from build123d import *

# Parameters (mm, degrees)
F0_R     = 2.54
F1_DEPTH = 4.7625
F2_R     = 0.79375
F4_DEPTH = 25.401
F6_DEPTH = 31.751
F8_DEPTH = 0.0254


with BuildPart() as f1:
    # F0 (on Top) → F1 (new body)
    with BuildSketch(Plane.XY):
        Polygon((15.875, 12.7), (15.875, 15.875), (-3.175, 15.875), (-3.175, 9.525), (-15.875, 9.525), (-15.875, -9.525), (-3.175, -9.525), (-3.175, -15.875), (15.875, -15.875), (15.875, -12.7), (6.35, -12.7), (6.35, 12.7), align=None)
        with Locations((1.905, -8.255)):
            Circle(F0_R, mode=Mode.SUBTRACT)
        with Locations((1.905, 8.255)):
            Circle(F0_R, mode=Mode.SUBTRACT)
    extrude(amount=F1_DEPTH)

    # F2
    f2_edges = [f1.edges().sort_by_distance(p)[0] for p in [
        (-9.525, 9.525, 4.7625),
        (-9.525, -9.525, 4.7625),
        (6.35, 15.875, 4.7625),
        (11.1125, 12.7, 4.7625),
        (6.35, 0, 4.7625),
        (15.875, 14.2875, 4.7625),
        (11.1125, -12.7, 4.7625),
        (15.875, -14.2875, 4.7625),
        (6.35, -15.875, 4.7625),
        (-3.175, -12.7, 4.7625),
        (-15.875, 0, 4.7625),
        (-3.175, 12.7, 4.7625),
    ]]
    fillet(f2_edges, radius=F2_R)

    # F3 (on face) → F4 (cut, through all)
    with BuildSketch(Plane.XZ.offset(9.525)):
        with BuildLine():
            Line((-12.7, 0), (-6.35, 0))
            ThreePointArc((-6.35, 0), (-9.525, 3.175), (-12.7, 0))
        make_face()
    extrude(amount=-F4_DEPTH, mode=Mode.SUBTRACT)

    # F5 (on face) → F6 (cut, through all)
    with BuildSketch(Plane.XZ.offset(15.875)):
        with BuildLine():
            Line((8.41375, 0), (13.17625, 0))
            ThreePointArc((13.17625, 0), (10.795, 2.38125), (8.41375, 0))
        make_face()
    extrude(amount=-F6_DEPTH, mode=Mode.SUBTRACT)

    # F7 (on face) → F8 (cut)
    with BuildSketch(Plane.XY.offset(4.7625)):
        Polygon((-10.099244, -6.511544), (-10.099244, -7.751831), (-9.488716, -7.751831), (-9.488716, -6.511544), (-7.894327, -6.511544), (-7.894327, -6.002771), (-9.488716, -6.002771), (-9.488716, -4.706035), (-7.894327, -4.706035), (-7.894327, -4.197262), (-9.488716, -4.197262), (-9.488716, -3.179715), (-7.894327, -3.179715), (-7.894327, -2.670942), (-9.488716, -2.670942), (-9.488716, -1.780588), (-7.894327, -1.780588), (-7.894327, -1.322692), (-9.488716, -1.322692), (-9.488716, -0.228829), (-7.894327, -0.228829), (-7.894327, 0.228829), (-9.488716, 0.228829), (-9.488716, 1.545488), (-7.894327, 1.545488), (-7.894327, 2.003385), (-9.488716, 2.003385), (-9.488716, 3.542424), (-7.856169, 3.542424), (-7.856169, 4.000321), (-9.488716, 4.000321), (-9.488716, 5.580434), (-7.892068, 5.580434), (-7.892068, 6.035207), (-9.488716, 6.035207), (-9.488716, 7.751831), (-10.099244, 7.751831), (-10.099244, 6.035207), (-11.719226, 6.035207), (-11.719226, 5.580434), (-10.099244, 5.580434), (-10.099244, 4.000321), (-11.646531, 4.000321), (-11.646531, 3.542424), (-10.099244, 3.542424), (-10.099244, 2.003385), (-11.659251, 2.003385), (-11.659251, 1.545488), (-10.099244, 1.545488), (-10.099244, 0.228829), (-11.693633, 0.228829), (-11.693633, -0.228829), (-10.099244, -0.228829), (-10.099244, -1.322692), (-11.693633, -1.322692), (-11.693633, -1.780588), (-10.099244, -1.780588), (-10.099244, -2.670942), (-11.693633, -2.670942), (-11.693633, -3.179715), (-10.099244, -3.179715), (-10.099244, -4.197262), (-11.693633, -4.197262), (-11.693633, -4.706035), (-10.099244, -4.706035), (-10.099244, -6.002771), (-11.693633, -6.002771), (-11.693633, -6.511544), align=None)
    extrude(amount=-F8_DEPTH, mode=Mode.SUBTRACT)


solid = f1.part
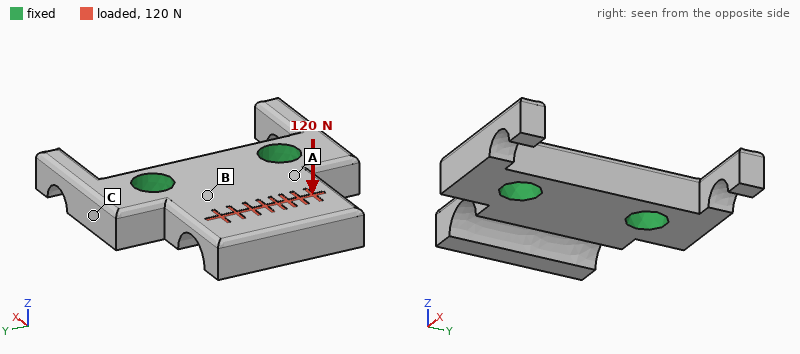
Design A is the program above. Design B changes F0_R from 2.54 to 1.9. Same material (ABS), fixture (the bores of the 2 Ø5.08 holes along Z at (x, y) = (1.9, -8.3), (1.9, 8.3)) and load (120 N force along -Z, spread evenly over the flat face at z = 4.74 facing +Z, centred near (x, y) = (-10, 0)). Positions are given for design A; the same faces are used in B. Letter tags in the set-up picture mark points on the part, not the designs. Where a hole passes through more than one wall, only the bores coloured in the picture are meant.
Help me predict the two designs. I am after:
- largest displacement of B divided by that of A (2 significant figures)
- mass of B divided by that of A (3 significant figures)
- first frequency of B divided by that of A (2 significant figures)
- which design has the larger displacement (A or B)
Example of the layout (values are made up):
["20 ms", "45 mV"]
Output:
["1.1", "1.04", "0.97", "B"]
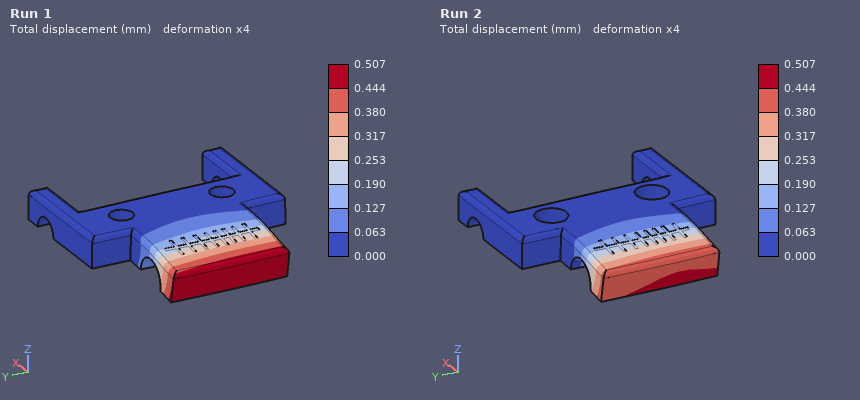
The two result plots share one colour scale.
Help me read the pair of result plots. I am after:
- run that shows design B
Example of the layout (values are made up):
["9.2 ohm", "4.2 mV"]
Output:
["Run 1"]
